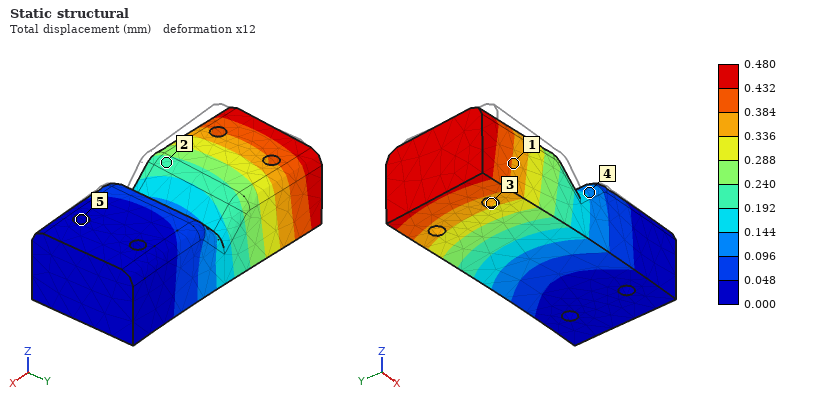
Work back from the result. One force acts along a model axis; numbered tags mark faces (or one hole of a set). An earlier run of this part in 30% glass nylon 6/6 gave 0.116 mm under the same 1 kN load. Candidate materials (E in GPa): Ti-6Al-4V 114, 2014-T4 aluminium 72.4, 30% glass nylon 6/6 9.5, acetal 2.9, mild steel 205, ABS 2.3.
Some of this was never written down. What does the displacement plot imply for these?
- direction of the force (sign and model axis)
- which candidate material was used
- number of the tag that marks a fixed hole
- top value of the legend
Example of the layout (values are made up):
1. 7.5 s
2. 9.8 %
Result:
1. +Y
2. ABS
3. 5
4. 0.480 mm
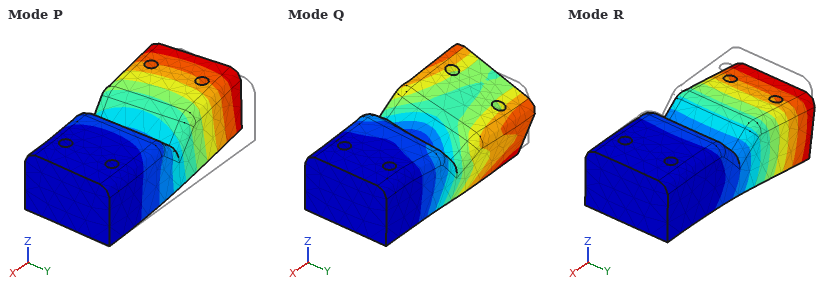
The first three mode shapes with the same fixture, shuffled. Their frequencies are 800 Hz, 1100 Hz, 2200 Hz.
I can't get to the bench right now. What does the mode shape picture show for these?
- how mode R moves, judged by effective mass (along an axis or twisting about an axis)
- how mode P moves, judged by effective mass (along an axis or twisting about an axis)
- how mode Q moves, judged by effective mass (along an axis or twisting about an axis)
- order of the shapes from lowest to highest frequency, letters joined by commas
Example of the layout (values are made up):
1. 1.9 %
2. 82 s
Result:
1. along Z
2. along Y
3. twisting about X
4. R, P, Q
